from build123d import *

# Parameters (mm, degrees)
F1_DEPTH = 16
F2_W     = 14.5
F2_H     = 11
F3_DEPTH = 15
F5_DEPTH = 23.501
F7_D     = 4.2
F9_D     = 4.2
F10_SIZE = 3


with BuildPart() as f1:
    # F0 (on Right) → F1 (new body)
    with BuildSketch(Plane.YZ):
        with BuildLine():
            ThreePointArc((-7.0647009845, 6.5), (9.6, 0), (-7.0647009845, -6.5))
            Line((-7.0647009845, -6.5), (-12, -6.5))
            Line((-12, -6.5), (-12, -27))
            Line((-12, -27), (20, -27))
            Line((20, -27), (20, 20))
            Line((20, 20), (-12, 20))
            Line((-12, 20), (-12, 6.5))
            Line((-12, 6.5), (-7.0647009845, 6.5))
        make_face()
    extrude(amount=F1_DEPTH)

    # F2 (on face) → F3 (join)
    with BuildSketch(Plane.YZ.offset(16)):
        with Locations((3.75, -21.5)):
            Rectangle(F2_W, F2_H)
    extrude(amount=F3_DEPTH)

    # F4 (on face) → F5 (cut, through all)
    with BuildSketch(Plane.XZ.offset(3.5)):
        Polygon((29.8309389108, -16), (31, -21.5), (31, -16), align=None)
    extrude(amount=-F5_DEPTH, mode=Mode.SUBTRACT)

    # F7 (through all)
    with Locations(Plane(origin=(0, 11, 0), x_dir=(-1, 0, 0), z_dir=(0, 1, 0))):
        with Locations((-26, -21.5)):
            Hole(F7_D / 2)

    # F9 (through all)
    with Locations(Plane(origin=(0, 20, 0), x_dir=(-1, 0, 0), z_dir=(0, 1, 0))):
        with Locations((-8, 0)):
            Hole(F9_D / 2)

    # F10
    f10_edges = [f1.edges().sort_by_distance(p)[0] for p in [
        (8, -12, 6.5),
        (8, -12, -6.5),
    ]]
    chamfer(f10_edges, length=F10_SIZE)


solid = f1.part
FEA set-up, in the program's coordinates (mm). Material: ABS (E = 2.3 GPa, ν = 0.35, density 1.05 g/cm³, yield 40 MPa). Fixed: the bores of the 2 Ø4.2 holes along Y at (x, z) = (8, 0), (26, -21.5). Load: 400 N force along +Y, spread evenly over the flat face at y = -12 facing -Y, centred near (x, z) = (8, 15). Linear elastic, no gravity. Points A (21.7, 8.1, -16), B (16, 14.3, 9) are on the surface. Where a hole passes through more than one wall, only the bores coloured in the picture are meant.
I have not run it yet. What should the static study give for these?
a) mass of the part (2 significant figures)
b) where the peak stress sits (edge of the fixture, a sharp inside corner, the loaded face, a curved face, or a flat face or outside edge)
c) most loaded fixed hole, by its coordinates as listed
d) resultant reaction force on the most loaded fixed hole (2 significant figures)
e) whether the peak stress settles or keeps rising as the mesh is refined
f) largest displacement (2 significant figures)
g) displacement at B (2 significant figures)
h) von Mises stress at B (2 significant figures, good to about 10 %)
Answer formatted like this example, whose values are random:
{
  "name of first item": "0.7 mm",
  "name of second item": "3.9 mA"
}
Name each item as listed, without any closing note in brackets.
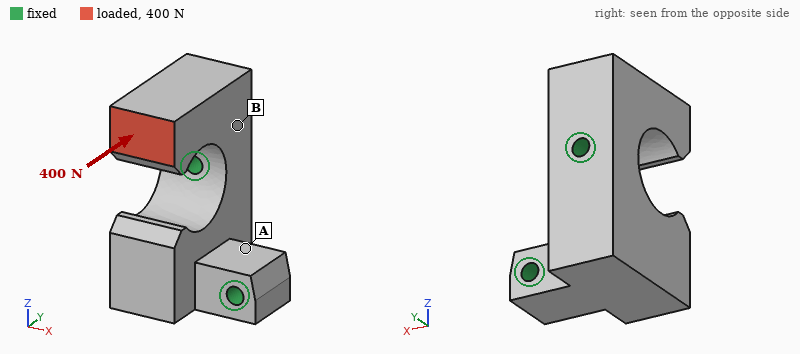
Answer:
{
  "mass of the part": "22 g",
  "where the peak stress sits": "edge of the fixture",
  "most loaded fixed hole, by its coordinates as listed": "(8, 0)",
  "resultant reaction force on the most loaded fixed hole": "430 N",
  "whether the peak stress settles or keeps rising as the mesh is refined": "keeps rising",
  "largest displacement": "0.39 mm",
  "displacement at B": "0.080 mm",
  "von Mises stress at B": "5.7 MPa"
}
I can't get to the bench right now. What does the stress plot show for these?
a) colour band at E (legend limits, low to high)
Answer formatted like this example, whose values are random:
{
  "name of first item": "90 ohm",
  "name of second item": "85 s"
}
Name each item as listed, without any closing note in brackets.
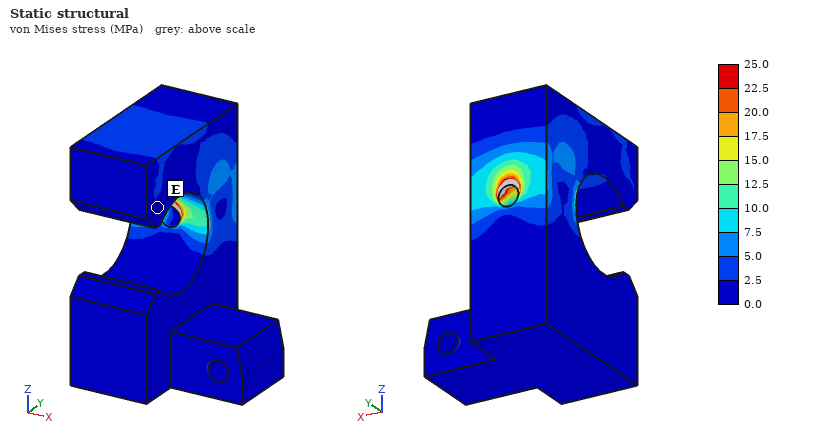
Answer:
{
  "colour band at E": "0.0 to 2.5 MPa"
}
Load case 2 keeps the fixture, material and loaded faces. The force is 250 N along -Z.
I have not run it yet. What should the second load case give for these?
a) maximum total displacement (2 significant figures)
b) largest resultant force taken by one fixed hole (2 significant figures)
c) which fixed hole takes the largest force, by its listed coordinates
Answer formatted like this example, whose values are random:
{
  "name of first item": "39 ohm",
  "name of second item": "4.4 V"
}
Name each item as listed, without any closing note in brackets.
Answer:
{
  "maximum total displacement": "0.77 mm",
  "largest resultant force taken by one fixed hole": "250 N",
  "which fixed hole takes the largest force, by its listed coordinates": "(8, 0)"
}
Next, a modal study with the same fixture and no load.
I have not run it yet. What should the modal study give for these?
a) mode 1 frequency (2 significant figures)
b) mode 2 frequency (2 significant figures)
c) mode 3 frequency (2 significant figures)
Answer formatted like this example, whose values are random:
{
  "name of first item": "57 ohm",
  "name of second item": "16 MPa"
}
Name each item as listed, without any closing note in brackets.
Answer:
{
  "mode 1 frequency": "2100 Hz",
  "mode 2 frequency": "2100 Hz",
  "mode 3 frequency": "2900 Hz"
}
